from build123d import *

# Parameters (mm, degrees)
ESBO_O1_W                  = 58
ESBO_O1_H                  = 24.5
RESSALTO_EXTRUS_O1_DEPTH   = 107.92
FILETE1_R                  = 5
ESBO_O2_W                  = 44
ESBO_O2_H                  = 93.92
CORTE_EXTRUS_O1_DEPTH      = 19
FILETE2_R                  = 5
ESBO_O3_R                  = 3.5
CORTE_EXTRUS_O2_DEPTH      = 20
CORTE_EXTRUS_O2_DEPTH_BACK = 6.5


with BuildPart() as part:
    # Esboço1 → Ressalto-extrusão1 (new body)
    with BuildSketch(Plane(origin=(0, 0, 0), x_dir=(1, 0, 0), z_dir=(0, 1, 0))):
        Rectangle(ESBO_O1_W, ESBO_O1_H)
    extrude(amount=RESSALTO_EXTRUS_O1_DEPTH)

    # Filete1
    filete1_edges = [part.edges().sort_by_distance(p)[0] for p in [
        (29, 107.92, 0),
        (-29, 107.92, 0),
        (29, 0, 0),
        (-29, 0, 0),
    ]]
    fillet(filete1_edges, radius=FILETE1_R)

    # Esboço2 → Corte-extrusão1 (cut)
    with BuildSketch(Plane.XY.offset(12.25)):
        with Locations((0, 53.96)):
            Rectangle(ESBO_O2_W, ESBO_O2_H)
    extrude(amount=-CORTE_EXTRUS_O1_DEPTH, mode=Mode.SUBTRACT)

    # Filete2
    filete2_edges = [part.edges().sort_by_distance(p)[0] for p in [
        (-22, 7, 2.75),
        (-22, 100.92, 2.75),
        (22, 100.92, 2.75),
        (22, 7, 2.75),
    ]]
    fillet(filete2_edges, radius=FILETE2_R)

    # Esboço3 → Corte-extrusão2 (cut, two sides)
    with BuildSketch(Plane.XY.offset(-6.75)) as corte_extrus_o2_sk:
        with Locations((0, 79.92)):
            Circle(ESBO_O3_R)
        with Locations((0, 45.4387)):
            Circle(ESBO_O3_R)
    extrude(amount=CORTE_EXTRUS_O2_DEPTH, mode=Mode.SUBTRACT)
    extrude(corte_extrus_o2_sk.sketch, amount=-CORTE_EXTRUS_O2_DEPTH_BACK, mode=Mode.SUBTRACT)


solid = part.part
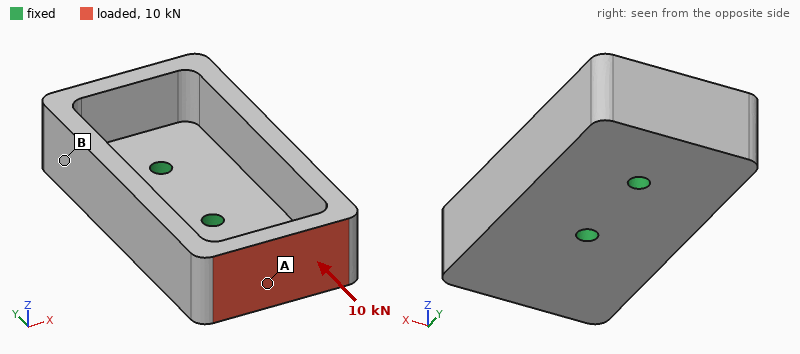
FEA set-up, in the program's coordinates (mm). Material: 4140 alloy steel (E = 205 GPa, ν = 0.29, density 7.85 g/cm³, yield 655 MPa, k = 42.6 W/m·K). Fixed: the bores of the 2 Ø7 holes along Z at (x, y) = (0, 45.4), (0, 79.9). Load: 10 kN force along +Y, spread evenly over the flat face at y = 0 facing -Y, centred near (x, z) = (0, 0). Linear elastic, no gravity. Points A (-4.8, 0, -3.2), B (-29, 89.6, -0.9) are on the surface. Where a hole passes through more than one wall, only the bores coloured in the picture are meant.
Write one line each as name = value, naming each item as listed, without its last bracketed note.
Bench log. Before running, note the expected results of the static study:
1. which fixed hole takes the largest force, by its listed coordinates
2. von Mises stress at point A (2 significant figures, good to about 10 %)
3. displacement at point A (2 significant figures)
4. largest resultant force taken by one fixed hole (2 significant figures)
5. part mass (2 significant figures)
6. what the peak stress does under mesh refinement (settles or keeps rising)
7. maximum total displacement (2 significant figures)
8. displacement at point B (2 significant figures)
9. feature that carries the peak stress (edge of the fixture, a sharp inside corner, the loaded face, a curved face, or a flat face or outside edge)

which fixed hole takes the largest force, by its listed coordinates = (0, 45.4)
von Mises stress at point A = 40 MPa
displacement at point A = 62 µm
largest resultant force taken by one fixed hole = 6.4 kN
part mass = 580 g
what the peak stress does under mesh refinement = keeps rising
maximum total displacement = 81 µm
displacement at point B = 18 µm
feature that carries the peak stress = edge of the fixture
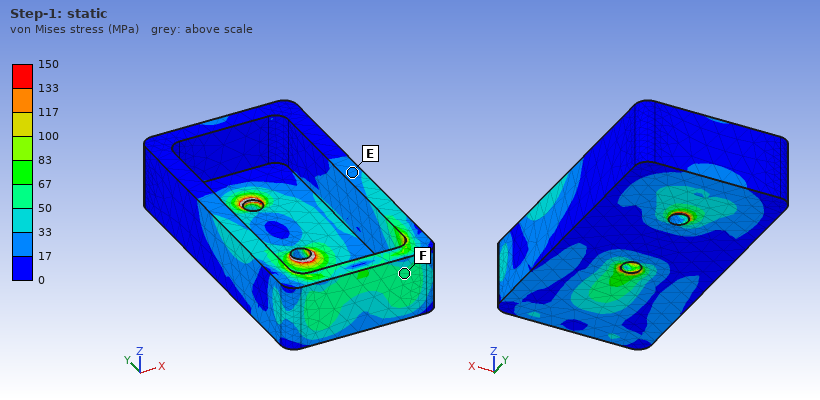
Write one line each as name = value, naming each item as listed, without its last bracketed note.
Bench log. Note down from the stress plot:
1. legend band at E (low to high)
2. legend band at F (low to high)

legend band at E = 17 to 33 MPa
legend band at F = 50 to 67 MPa
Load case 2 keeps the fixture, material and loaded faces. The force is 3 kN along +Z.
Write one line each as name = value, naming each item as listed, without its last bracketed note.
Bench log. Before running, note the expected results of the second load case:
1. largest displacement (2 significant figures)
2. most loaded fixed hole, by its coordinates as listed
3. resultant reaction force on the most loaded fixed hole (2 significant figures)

largest displacement = 0.13 mm
most loaded fixed hole, by its coordinates as listed = (0, 45.4)
resultant reaction force on the most loaded fixed hole = 5.6 kN
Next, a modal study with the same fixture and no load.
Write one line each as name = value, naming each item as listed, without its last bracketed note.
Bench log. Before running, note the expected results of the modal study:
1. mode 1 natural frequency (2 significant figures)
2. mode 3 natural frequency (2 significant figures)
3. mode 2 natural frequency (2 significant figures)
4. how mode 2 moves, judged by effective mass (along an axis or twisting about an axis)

mode 1 natural frequency = 1800 Hz
mode 3 natural frequency = 2900 Hz
mode 2 natural frequency = 2000 Hz
how mode 2 moves, judged by effective mass = along Z
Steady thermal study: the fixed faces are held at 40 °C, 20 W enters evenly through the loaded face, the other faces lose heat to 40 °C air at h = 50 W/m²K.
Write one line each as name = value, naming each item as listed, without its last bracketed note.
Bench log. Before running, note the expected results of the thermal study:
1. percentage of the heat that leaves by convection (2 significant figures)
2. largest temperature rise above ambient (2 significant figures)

percentage of the heat that leaves by convection = 57 %
largest temperature rise above ambient = 36 K
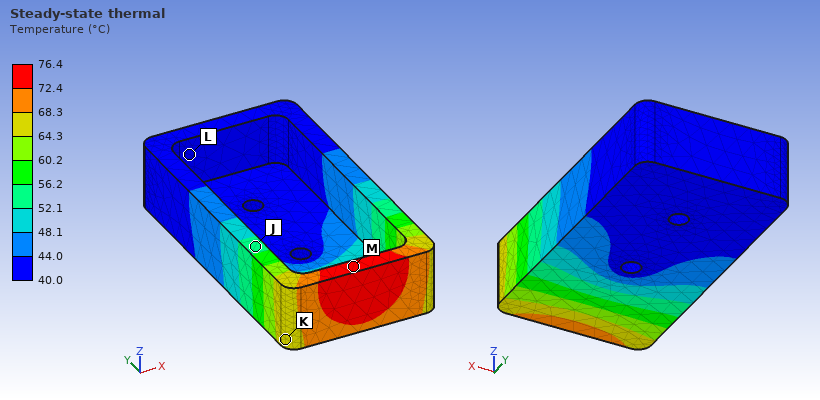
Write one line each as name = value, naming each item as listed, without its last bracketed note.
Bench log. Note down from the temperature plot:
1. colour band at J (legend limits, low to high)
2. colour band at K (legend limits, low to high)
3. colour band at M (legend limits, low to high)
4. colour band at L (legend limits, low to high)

colour band at J = 52.1 to 56.2 °C
colour band at K = 64.3 to 68.3 °C
colour band at M = 72.4 to 76.4 °C
colour band at L = 40.0 to 44.0 °C
